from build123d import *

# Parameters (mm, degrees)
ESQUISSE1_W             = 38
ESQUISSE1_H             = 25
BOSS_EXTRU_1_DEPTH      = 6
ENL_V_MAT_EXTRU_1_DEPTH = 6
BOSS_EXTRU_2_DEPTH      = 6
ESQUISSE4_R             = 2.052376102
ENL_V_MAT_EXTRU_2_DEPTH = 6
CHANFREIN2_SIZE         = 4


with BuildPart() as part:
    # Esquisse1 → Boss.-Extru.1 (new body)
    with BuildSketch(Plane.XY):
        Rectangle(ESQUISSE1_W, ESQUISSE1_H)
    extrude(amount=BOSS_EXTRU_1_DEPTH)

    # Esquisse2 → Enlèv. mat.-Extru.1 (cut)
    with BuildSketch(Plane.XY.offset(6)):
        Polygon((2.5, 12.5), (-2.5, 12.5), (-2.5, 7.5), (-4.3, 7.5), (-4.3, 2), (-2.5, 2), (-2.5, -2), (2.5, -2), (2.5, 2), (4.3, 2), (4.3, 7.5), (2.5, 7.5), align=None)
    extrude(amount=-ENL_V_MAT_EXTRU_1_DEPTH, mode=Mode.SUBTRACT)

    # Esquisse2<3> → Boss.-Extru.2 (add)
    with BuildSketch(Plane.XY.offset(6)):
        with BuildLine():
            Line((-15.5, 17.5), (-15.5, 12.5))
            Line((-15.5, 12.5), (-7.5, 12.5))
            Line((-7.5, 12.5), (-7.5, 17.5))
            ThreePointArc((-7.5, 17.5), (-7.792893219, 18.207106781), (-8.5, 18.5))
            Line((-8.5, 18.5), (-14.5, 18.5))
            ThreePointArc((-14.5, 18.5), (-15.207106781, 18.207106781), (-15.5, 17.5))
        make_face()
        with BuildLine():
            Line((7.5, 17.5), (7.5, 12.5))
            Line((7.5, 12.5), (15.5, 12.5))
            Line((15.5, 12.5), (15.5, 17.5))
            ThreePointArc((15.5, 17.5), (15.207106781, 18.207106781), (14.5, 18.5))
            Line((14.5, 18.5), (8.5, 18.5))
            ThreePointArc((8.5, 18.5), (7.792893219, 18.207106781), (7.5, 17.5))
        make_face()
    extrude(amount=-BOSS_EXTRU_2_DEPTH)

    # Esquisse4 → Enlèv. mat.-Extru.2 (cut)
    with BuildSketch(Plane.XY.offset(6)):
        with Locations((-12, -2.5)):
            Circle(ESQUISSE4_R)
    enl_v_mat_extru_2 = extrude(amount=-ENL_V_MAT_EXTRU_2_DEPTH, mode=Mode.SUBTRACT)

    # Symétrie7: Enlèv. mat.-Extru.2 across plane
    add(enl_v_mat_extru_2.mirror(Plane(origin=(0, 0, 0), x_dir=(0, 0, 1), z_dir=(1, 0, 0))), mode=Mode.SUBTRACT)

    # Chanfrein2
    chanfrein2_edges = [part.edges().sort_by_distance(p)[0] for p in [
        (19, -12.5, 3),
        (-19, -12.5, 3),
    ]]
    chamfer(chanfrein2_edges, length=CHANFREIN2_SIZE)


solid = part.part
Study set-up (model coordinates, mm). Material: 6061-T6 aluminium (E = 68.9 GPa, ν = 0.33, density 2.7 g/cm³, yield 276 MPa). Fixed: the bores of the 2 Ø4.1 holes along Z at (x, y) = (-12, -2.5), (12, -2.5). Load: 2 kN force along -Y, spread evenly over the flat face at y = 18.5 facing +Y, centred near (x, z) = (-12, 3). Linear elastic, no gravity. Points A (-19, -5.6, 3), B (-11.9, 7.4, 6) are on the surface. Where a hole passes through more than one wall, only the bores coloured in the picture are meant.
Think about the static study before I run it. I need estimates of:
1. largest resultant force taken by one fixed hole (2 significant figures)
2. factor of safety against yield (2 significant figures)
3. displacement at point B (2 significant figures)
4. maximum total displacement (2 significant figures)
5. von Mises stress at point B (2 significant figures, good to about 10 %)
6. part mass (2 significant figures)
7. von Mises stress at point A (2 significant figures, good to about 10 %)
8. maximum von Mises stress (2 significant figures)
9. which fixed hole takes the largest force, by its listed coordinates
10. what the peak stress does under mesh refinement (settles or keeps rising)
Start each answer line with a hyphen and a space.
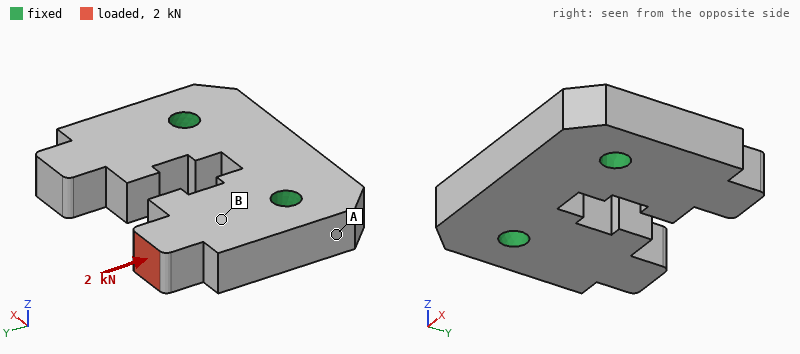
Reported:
- 1.9 kN
- 4.3
- 4.0 µm
- 11 µm
- 35 MPa
- 15 g
- 7.6 MPa
- 65 MPa
- (-12, -2.5)
- settles
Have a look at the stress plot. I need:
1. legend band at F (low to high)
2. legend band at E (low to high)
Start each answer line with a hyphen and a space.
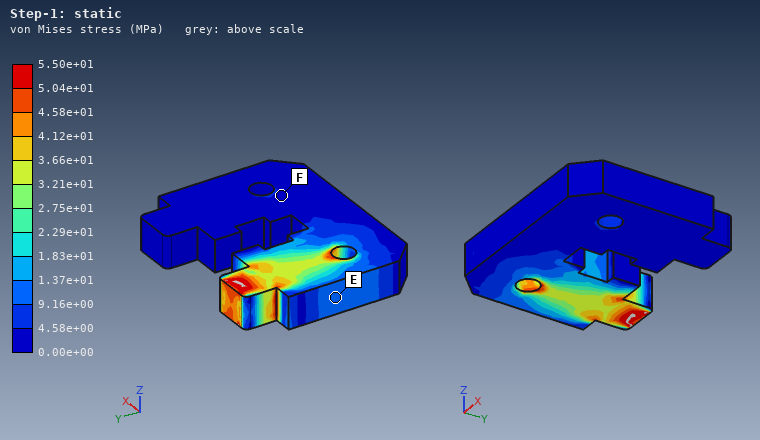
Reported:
- 0.00e+00 to 4.58e+00 MPa
- 9.16e+00 to 1.37e+01 MPa
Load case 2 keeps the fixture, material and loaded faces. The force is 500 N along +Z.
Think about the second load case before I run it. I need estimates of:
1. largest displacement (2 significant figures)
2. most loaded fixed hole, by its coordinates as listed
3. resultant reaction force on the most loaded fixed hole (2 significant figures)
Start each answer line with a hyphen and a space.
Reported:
- 94 µm
- (-12, -2.5)
- 550 N
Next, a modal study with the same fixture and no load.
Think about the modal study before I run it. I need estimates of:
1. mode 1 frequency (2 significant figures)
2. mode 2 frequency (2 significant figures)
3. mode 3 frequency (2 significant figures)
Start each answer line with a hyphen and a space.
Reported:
- 13 kHz
- 13 kHz
- 19 kHz
